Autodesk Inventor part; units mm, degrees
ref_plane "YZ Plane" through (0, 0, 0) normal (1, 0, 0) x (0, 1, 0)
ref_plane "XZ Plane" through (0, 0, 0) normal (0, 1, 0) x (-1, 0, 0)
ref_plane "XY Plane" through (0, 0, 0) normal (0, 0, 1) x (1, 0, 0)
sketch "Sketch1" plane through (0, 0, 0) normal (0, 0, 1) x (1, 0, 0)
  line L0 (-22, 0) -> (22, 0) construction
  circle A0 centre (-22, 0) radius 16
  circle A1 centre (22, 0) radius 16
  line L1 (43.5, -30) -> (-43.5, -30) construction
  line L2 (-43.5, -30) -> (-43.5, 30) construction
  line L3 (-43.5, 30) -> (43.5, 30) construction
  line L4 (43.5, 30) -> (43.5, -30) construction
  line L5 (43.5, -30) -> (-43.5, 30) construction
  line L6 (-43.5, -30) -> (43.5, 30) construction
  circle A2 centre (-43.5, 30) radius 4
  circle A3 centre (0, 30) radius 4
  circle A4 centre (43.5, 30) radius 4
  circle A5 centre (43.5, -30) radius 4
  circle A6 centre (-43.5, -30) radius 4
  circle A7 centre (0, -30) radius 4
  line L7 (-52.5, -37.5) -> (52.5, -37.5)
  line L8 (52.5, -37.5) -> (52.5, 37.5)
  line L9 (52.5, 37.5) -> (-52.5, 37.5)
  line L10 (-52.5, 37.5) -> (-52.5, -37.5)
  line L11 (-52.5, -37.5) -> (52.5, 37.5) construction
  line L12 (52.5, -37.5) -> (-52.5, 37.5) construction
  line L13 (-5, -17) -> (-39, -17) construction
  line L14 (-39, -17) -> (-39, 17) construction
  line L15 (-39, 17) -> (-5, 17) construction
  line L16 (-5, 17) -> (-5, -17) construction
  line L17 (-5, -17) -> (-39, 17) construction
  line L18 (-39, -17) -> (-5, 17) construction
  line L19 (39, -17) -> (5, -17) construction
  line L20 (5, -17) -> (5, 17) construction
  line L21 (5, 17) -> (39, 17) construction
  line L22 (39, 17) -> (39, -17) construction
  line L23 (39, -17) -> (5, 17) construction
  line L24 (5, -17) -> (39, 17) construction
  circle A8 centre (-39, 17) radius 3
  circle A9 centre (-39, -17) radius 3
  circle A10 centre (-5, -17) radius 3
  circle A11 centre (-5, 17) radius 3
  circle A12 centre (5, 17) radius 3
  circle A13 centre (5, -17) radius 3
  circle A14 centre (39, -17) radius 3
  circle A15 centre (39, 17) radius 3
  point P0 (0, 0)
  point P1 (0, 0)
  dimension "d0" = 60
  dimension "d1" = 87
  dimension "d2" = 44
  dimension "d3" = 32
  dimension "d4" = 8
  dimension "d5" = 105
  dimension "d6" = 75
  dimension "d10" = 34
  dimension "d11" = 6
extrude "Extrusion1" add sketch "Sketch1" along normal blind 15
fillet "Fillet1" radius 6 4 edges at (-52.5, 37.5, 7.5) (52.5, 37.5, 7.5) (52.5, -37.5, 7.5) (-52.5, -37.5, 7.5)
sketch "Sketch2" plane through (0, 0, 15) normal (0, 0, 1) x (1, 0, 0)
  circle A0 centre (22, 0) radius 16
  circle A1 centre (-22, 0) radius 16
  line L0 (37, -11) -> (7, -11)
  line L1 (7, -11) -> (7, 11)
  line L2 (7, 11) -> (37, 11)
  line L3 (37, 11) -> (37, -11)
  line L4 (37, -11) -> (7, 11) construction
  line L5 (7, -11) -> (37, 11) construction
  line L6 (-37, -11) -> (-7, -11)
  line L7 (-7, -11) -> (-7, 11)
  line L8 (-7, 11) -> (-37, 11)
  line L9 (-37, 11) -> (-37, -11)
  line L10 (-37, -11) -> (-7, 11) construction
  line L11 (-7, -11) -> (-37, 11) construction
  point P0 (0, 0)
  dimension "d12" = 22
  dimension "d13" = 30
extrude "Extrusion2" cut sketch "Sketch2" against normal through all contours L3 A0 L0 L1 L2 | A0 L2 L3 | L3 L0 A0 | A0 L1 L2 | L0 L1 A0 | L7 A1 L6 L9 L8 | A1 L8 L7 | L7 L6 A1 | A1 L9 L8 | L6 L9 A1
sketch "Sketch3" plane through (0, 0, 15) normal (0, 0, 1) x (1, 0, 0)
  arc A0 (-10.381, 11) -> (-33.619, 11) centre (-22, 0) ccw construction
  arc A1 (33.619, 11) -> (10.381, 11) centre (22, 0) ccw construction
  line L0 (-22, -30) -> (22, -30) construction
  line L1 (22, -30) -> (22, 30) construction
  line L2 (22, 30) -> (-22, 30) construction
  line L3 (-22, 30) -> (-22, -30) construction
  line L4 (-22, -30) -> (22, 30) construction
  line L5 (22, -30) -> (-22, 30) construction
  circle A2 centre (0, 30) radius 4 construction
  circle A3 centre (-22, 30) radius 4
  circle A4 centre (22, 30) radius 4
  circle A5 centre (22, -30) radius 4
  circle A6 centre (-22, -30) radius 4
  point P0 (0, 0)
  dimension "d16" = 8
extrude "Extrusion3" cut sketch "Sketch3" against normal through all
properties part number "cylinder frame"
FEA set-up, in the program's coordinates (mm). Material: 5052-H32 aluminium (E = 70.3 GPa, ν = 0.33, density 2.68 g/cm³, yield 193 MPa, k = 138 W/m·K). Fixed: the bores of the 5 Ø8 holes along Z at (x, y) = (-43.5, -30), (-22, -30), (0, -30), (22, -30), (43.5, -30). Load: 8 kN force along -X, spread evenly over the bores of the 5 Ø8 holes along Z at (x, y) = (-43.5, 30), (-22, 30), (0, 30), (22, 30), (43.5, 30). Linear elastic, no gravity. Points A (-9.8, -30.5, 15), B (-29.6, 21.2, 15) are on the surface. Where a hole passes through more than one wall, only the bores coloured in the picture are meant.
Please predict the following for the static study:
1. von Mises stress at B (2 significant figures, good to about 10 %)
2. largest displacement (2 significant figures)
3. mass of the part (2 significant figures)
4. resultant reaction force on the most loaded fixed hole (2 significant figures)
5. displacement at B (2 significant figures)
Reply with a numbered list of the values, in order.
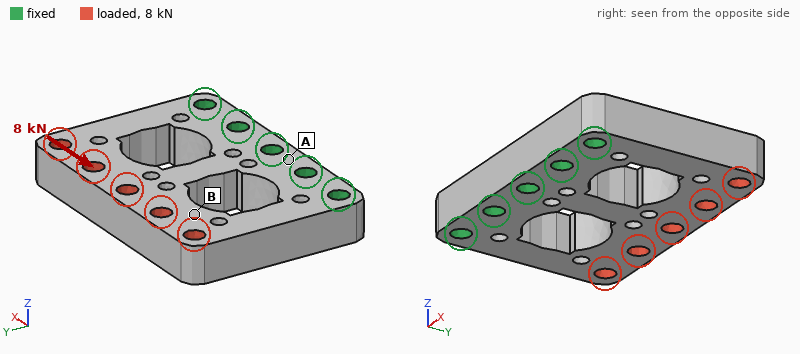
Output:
1. 18 MPa
2. 81 µm
3. 220 g
4. 5.1 kN
5. 68 µm
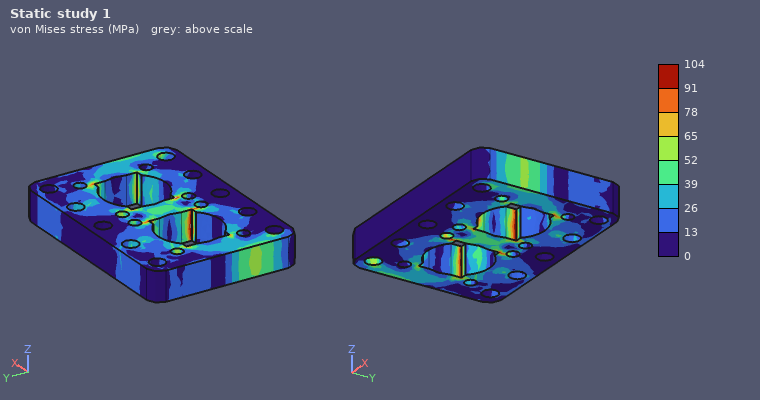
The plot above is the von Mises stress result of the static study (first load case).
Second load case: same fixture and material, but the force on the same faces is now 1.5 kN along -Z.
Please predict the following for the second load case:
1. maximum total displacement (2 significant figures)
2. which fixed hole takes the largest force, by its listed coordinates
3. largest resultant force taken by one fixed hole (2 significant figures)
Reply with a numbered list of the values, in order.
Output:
1. 0.14 mm
2. (0, -30)
3. 380 N
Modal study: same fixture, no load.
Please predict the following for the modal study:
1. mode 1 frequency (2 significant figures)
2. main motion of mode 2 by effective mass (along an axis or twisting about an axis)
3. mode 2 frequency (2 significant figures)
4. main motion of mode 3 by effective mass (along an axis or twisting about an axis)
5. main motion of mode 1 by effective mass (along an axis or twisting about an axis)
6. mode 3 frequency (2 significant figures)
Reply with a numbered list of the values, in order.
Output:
1. 2100 Hz
2. twisting about Y
3. 3700 Hz
4. along X
5. along Z
6. 5400 Hz
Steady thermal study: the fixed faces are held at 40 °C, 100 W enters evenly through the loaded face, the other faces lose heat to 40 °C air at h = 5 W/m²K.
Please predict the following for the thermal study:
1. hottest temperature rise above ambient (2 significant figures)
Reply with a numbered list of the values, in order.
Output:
1. 58 K
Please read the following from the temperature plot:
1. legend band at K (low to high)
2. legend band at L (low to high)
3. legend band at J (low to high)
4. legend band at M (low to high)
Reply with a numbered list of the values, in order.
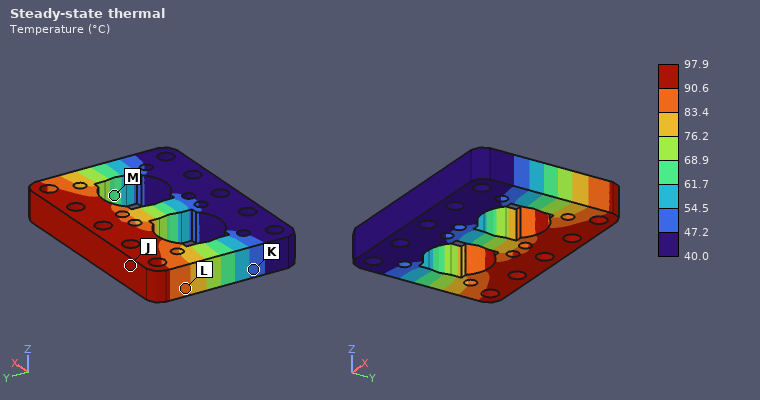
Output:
1. 47.2 to 54.5 °C
2. 83.4 to 90.6 °C
3. 90.6 to 97.9 °C
4. 61.7 to 68.9 °C
